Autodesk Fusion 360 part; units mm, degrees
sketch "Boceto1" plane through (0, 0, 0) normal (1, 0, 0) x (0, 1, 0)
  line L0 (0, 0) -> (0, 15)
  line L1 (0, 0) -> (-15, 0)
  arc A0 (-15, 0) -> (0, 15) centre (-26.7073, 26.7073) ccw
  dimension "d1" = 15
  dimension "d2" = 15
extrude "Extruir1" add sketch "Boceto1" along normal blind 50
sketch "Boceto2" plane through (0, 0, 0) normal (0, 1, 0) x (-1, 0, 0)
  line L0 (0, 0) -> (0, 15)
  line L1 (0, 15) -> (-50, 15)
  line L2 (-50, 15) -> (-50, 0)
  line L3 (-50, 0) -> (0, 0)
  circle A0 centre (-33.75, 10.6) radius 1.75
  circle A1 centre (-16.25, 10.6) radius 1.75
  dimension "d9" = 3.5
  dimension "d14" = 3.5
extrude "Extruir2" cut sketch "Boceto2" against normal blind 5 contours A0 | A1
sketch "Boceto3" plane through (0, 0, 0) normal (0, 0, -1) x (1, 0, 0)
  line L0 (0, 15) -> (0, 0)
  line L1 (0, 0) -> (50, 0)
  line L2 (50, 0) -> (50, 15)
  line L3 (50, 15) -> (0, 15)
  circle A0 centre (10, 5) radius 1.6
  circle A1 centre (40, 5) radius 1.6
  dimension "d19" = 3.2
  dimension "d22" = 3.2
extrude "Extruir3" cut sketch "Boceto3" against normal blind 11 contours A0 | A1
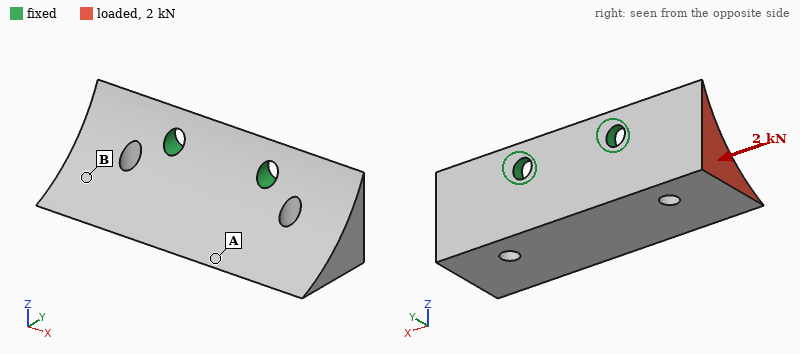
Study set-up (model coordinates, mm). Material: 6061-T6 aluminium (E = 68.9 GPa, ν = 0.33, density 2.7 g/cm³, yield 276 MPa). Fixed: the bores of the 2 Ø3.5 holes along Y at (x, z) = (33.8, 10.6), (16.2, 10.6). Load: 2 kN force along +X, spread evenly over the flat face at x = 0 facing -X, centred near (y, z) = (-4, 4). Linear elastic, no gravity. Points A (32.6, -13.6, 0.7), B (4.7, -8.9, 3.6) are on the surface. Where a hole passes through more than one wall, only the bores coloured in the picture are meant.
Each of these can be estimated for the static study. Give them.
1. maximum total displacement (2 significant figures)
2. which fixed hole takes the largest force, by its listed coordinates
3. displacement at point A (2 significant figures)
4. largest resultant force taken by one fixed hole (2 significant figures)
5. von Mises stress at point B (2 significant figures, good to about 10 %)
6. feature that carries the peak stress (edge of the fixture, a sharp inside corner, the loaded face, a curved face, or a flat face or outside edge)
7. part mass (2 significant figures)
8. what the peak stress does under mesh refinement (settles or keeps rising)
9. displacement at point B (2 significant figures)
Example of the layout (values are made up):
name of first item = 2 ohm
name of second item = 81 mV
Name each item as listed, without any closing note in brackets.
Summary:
maximum total displacement = 23 µm
which fixed hole takes the largest force, by its listed coordinates = (16.2, 10.6)
displacement at point A = 8.6 µm
largest resultant force taken by one fixed hole = 1.4 kN
von Mises stress at point B = 28 MPa
feature that carries the peak stress = edge of the fixture
part mass = 11 g
what the peak stress does under mesh refinement = keeps rising
displacement at point B = 16 µm
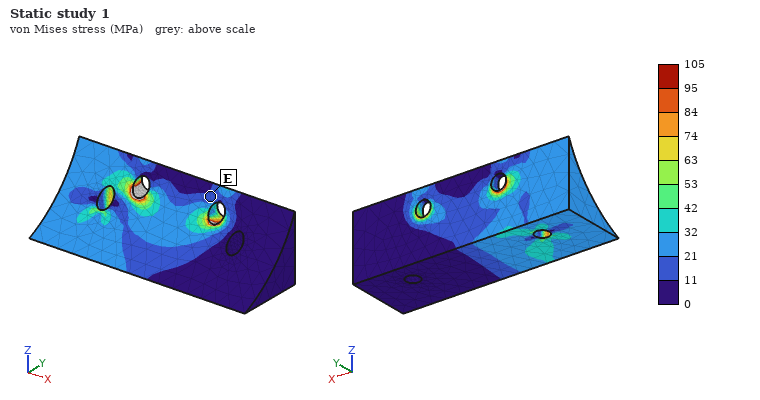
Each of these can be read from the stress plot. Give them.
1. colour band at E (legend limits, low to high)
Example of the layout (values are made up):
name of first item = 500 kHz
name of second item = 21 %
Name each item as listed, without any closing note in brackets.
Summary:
colour band at E = 11 to 21 MPa
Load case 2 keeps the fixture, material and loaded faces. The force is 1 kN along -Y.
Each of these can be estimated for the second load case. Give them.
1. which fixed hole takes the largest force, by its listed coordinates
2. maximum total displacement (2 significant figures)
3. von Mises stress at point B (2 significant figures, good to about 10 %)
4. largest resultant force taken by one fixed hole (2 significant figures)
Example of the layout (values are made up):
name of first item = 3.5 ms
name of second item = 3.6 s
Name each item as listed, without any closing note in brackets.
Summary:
which fixed hole takes the largest force, by its listed coordinates = (16.2, 10.6)
maximum total displacement = 0.20 mm
von Mises stress at point B = 51 MPa
largest resultant force taken by one fixed hole = 1.7 kN
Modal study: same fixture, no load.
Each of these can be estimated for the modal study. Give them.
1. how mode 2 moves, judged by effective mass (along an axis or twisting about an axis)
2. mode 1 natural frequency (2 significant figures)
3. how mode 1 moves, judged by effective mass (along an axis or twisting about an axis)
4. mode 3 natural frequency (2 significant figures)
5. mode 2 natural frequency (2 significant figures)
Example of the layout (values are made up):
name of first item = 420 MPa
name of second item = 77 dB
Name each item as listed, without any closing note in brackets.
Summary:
how mode 2 moves, judged by effective mass = twisting about Z
mode 1 natural frequency = 8400 Hz
how mode 1 moves, judged by effective mass = along Y
mode 3 natural frequency = 15 kHz
mode 2 natural frequency = 9300 Hz
